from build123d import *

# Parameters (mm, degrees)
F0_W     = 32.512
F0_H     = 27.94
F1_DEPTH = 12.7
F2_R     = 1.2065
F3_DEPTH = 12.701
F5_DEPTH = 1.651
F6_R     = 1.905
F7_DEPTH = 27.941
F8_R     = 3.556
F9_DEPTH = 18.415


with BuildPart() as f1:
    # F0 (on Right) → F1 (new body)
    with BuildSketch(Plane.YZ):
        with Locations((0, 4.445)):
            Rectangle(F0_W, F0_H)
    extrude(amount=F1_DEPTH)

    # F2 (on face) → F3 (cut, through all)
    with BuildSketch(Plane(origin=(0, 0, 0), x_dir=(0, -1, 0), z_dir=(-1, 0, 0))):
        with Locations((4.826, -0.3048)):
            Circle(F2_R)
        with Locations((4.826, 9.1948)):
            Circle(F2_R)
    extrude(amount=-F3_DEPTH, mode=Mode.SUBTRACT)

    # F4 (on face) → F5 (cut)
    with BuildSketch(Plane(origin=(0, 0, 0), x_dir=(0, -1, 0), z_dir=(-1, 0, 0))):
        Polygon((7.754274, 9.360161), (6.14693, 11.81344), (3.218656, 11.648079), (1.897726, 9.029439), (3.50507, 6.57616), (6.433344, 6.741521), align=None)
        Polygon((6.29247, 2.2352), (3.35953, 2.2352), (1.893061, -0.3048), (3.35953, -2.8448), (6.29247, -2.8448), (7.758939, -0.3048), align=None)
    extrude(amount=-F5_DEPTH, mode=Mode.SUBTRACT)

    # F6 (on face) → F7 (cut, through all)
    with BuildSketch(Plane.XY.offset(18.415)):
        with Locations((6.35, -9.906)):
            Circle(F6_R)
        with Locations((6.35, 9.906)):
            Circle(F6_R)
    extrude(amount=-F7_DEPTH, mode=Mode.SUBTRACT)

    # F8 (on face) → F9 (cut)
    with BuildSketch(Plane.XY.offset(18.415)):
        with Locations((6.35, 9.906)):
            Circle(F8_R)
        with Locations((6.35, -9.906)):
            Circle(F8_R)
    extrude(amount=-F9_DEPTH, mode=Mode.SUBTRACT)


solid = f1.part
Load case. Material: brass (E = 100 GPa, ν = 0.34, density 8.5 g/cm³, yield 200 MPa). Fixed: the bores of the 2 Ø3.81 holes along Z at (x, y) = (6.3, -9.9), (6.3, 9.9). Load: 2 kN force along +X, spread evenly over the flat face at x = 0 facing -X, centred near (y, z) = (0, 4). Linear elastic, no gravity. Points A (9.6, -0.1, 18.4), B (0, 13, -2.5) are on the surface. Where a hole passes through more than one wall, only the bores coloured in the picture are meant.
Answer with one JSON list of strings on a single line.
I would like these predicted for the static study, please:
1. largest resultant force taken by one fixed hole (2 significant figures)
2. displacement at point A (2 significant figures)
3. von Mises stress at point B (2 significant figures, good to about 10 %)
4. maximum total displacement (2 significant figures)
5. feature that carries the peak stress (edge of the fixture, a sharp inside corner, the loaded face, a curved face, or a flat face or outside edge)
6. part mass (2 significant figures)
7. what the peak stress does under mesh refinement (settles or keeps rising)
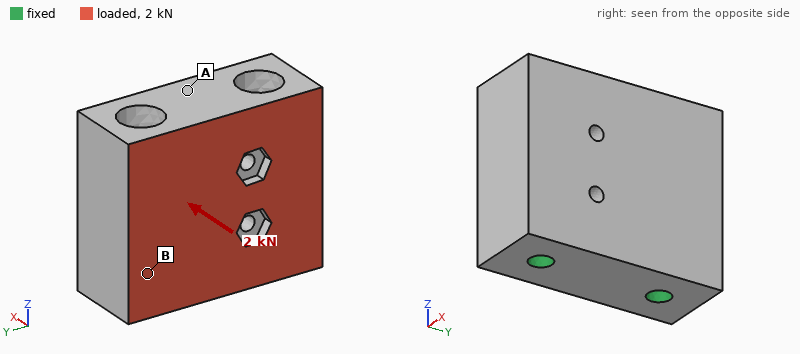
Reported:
["1.0 kN", "13 µm", "22 MPa", "14 µm", "edge of the fixture", "82 g", "keeps rising"]
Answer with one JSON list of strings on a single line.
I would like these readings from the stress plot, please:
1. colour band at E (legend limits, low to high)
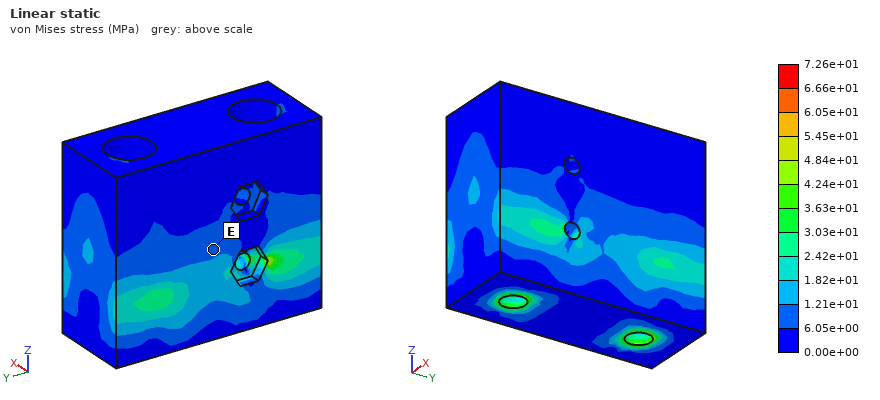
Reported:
["6.05e+00 to 1.21e+01 MPa"]
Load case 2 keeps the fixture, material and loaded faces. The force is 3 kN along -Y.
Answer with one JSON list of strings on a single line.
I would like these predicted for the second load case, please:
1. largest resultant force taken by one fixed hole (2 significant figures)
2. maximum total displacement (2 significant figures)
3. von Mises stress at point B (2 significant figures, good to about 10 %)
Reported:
["2.0 kN", "9.7 µm", "11 MPa"]
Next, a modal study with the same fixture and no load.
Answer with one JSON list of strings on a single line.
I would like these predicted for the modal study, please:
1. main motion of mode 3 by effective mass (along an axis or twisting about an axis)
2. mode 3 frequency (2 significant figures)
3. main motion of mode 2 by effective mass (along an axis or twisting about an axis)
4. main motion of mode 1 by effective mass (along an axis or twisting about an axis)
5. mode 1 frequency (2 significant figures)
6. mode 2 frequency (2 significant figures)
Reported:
["twisting about Z", "16 kHz", "along Y", "along X", "8300 Hz", "15 kHz"]
